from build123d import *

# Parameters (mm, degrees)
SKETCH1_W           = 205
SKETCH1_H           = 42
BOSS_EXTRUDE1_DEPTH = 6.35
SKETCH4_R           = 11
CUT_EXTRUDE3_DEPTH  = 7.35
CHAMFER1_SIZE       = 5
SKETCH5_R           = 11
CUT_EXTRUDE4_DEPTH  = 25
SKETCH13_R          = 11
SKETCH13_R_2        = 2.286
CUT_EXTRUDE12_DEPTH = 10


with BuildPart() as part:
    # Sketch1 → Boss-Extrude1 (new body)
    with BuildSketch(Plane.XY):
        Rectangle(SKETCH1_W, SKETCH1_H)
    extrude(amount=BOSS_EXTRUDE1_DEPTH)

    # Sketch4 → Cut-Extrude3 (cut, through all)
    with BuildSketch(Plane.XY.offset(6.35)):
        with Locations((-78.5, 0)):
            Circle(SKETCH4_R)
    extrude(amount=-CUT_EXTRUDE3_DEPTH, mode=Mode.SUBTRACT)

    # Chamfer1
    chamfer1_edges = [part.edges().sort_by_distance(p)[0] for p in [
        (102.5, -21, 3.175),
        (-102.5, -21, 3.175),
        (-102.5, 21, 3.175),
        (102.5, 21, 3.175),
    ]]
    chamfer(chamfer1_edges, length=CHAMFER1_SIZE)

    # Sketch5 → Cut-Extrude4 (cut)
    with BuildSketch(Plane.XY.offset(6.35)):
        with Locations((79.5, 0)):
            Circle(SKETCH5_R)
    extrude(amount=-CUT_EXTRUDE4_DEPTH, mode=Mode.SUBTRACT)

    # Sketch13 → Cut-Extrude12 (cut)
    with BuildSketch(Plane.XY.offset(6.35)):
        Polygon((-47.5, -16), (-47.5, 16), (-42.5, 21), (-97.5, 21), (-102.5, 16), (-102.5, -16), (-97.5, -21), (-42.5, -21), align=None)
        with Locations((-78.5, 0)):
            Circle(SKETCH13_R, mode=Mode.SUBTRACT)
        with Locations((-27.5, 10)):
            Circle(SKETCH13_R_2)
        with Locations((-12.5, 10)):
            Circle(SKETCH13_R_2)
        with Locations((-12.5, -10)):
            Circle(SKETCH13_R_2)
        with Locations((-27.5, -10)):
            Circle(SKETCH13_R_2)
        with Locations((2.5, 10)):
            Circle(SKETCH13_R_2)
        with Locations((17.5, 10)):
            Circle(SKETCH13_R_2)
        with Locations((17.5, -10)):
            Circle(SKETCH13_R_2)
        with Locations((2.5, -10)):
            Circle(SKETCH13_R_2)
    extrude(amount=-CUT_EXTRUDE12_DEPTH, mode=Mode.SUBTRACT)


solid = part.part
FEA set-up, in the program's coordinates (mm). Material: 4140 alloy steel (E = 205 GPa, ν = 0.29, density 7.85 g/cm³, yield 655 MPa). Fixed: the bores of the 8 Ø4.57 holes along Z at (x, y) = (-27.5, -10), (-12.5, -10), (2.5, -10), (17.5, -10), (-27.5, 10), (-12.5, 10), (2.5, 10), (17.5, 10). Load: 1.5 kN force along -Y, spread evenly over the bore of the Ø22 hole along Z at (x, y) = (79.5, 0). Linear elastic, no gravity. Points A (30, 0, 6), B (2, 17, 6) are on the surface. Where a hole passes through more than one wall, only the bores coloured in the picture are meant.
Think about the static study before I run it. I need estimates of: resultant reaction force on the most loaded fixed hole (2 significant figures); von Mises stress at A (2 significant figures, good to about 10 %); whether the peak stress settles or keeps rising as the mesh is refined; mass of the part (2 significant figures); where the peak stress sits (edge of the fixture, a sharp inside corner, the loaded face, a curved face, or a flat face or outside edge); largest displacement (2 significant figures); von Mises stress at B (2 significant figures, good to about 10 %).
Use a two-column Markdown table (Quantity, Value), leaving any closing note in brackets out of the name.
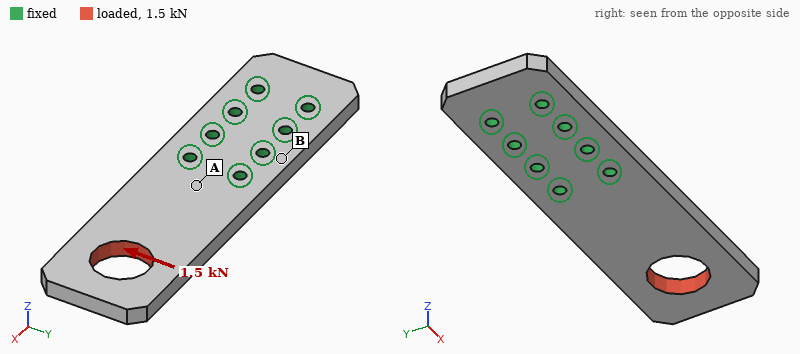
| Quantity | Value |
|---|---|
| resultant reaction force on the most loaded fixed hole | 2.9 kN |
| von Mises stress at A | 19 MPa |
| whether the peak stress settles or keeps rising as the mesh is refined | keeps rising |
| mass of the part | 290 g |
| where the peak stress sits | edge of the fixture |
| largest displacement | 39 µm |
| von Mises stress at B | 7.7 MPa |
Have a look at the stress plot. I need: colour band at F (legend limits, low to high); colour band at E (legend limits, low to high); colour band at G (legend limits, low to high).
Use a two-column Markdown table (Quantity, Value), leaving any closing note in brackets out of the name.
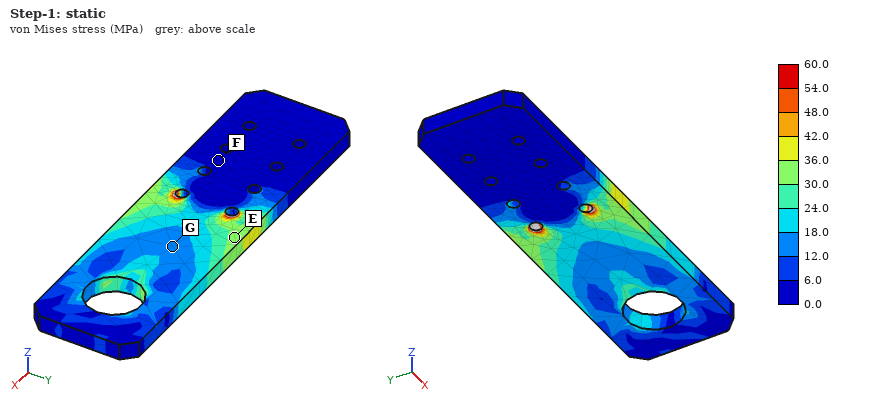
| Quantity | Value |
|---|---|
| colour band at F | 0.0 to 6.0 MPa |
| colour band at E | 30.0 to 36.0 MPa |
| colour band at G | 12.0 to 18.0 MPa |
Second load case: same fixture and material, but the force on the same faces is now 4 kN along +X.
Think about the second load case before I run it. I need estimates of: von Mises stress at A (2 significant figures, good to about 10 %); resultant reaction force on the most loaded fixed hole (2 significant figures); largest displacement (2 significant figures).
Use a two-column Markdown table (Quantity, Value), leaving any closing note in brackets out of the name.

| Quantity | Value |
|---|---|
| von Mises stress at A | 14 MPa |
| resultant reaction force on the most loaded fixed hole | 1.6 kN |
| largest displacement | 8.0 µm |
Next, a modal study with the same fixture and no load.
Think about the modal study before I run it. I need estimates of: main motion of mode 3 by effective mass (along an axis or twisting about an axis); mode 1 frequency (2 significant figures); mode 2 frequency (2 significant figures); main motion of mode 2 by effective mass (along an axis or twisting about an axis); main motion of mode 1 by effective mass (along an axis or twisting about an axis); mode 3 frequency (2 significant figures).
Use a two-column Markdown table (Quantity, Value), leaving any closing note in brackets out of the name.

| Quantity | Value |
|---|---|
| main motion of mode 3 by effective mass | along Y |
| mode 1 frequency | 810 Hz |
| mode 2 frequency | 2900 Hz |
| main motion of mode 2 by effective mass | twisting about X |
| main motion of mode 1 by effective mass | along Z |
| mode 3 frequency | 4000 Hz |
